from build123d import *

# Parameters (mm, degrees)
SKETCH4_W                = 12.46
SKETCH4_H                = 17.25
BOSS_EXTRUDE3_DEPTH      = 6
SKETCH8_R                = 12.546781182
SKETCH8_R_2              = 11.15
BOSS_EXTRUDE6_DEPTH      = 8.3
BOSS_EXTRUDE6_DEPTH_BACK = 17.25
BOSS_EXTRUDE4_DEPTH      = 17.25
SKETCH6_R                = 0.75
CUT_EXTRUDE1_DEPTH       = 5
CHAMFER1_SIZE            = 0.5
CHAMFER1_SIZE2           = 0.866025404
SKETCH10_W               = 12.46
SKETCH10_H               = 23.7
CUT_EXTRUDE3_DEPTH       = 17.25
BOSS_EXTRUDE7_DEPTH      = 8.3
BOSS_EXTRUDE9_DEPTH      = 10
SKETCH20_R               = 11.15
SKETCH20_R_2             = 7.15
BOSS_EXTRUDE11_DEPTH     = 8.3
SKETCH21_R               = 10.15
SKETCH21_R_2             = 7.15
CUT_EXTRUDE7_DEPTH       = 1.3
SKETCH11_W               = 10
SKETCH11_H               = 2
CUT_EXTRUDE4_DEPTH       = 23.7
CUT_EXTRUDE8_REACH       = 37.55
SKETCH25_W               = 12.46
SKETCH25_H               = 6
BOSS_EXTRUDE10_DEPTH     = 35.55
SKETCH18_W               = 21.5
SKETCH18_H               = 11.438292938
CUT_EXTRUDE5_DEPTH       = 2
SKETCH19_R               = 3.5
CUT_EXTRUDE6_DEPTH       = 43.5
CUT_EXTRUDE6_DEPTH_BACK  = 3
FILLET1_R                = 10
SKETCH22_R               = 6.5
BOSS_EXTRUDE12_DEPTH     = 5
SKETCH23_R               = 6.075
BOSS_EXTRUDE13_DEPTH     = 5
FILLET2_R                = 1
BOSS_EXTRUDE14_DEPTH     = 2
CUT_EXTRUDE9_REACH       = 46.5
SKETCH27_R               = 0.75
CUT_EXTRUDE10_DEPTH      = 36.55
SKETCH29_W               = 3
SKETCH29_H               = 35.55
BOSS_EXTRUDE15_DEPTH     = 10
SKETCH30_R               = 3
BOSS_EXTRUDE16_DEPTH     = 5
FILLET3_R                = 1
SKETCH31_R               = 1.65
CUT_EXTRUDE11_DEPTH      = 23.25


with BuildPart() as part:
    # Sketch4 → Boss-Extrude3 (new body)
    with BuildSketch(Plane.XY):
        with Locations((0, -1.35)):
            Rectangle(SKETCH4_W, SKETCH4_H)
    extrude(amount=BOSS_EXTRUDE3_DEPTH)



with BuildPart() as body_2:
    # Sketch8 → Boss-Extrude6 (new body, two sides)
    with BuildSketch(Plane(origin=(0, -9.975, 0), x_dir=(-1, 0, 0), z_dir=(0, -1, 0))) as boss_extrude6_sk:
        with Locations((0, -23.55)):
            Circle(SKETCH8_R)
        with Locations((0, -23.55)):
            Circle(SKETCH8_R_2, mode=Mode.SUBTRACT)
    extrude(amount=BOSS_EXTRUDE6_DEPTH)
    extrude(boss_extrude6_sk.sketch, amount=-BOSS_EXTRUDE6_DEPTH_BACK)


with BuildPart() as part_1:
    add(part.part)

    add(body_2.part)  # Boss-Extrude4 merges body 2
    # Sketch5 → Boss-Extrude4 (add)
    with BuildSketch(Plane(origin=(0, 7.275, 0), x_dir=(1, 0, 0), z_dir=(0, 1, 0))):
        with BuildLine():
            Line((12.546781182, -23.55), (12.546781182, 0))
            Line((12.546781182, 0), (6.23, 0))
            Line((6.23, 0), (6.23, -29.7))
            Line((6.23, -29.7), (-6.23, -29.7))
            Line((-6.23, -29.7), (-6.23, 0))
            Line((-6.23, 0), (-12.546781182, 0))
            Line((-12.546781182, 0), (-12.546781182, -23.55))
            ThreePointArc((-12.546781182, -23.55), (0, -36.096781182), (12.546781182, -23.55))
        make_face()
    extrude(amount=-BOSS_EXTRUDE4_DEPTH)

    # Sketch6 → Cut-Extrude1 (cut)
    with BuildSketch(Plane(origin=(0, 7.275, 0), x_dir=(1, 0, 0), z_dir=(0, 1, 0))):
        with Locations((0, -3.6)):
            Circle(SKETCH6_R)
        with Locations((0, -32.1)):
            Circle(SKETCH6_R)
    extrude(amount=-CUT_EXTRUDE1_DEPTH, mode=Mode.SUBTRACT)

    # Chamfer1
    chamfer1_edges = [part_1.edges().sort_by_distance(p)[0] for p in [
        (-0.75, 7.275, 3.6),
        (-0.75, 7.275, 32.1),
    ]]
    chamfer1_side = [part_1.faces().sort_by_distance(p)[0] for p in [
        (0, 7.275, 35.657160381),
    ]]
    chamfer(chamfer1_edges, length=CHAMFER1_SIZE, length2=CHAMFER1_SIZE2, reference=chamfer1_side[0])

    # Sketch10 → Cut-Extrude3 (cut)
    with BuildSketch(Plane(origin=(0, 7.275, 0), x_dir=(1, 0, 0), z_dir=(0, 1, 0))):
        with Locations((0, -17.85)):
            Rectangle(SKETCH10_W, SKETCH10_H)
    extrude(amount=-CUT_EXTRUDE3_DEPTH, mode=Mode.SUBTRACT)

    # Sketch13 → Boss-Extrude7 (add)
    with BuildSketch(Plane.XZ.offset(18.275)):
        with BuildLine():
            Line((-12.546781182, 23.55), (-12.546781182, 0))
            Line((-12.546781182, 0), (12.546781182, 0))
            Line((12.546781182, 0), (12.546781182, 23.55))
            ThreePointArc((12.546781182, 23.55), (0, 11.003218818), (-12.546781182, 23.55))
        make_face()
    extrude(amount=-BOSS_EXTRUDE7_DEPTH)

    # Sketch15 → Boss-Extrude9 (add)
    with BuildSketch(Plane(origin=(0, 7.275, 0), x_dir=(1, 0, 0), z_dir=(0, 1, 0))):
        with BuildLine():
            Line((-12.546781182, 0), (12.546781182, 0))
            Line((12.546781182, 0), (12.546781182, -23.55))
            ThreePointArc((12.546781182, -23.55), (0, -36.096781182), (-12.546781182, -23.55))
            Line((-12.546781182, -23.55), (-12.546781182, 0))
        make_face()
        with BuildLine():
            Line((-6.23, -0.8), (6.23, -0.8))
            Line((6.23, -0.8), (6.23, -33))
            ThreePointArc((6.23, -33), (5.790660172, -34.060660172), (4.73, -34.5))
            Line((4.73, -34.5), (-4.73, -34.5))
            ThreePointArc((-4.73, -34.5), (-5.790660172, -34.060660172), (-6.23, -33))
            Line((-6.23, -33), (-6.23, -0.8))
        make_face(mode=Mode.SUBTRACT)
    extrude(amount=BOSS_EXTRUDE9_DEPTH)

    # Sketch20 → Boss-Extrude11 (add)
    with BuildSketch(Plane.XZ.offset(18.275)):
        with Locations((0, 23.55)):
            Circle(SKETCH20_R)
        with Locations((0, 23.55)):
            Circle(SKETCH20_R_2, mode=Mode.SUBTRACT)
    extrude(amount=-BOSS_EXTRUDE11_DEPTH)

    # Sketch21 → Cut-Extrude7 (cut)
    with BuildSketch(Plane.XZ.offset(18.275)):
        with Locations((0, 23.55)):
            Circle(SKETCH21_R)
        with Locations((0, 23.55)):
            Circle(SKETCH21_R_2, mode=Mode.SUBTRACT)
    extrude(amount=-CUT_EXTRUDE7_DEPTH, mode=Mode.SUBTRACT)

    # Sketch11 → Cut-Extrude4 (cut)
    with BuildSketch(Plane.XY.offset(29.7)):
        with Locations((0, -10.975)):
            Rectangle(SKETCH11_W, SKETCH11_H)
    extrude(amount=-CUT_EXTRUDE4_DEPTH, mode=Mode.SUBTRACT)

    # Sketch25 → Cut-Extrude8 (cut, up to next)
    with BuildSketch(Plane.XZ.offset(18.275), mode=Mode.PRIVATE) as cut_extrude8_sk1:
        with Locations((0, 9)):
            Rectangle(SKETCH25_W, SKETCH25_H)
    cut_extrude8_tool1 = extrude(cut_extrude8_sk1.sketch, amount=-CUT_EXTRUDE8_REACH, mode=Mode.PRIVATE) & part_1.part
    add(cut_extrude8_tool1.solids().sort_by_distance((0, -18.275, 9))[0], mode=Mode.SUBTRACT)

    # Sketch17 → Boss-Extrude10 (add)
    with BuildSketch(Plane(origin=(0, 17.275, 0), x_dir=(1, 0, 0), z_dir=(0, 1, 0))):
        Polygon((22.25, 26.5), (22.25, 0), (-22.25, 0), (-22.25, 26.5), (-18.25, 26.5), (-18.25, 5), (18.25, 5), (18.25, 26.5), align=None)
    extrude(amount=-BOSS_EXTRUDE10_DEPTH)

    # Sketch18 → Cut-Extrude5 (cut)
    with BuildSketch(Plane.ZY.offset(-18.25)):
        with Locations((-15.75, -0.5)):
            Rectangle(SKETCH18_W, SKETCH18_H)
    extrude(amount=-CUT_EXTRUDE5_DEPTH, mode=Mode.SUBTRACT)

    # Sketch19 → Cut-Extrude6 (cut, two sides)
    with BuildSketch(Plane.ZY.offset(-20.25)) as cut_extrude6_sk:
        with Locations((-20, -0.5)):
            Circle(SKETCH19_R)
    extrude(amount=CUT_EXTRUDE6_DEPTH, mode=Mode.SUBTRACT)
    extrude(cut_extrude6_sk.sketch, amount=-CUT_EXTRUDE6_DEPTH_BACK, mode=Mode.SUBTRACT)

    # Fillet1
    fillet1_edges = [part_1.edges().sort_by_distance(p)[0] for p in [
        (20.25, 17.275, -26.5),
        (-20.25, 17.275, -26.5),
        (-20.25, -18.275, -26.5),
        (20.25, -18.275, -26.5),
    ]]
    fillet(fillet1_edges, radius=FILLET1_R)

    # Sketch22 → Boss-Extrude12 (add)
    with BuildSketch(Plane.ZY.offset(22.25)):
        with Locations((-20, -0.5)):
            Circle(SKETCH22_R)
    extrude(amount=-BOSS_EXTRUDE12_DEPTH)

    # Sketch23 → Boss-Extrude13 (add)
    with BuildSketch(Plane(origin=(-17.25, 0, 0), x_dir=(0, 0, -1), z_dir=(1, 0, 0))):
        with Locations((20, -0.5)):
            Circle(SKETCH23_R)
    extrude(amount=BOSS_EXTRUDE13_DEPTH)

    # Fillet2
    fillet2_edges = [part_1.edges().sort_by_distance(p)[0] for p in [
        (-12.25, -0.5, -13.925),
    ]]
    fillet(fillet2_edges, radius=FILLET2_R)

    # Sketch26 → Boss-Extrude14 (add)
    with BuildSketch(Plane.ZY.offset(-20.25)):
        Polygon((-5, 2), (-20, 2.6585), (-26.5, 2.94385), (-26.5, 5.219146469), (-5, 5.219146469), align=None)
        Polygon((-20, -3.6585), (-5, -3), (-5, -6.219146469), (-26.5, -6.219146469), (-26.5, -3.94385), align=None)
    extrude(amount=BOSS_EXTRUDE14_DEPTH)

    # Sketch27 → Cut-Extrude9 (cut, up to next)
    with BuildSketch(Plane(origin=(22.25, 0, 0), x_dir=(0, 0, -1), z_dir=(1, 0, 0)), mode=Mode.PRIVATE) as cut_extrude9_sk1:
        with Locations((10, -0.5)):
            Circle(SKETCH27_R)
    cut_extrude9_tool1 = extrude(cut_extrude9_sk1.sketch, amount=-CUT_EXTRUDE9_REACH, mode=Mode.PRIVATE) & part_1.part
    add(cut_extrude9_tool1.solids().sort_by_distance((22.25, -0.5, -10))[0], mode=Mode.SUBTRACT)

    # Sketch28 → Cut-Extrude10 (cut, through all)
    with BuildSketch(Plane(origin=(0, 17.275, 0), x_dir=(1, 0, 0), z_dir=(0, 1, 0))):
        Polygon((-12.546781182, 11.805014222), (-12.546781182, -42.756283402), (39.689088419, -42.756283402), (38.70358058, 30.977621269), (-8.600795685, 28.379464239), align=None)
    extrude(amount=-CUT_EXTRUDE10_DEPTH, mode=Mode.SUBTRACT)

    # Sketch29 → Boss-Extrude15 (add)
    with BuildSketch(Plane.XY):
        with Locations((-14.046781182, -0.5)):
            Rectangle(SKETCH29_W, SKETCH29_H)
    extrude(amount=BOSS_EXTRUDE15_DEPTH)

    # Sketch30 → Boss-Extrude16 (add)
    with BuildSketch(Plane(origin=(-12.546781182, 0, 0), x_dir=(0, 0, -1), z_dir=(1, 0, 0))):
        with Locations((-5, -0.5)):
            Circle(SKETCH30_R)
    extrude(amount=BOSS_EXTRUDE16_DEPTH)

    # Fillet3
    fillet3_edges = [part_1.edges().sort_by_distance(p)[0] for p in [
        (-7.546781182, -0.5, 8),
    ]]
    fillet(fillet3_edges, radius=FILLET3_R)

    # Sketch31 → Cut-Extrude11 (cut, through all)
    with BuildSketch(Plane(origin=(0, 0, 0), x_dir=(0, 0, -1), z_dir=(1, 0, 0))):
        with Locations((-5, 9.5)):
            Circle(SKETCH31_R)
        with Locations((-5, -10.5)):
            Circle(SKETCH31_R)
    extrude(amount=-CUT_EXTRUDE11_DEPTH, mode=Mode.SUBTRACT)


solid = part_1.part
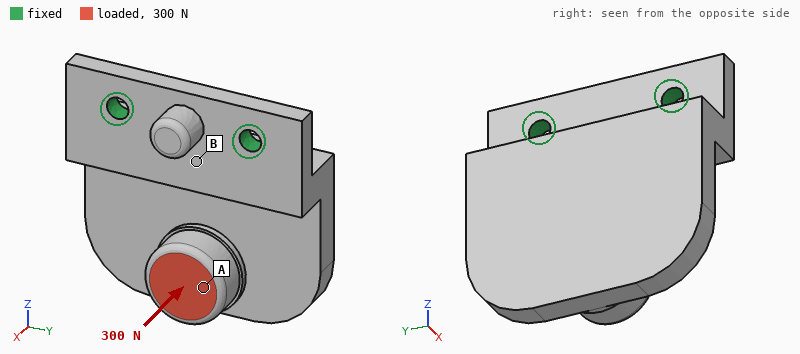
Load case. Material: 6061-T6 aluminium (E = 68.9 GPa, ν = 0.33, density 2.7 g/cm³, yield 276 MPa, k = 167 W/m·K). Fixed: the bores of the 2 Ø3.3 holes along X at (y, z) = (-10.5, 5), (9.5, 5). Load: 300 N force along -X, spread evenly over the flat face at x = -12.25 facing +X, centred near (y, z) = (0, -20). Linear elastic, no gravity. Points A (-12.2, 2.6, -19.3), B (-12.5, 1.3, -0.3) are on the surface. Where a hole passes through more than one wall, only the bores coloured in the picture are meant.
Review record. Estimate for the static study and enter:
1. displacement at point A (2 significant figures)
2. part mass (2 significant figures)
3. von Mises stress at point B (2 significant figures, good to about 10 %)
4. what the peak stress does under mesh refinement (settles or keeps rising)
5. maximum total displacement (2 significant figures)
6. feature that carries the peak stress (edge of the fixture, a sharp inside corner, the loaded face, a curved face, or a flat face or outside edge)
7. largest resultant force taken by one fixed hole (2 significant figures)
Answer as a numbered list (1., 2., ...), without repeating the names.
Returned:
1. 0.22 mm
2. 17 g
3. 76 MPa
4. keeps rising
5. 0.30 mm
6. edge of the fixture
7. 150 N
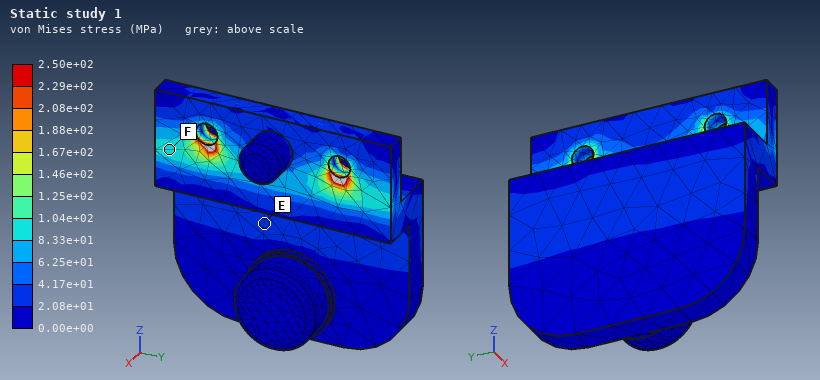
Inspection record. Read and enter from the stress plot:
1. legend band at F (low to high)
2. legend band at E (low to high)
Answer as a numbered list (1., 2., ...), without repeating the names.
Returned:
1. 8.33e+01 to 1.04e+02 MPa
2. 2.08e+01 to 4.17e+01 MPa
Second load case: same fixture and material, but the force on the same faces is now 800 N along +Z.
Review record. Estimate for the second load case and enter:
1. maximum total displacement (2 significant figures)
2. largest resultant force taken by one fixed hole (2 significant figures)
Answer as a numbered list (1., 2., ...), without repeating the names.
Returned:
1. 0.18 mm
2. 400 N
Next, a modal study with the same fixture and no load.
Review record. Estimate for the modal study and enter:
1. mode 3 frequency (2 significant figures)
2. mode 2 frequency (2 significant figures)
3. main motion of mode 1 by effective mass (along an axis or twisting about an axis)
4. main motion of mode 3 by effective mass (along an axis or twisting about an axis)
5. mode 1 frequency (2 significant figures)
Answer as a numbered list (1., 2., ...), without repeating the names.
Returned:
1. 11 kHz
2. 6600 Hz
3. along X
4. along Y
5. 2100 Hz
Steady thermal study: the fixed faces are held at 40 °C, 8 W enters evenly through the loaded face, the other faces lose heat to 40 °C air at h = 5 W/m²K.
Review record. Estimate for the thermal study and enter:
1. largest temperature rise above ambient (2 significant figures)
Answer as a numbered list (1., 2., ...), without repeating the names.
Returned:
1. 14 K
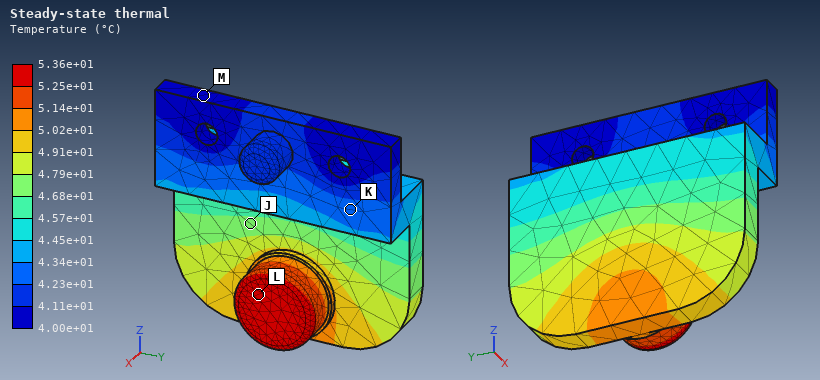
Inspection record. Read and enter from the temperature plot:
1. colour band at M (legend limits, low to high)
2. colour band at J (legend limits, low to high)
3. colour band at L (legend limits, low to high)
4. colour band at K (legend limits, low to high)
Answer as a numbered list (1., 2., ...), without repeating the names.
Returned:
1. 4.00e+01 to 4.11e+01 °C
2. 4.68e+01 to 4.79e+01 °C
3. 5.25e+01 to 5.36e+01 °C
4. 4.23e+01 to 4.34e+01 °C
